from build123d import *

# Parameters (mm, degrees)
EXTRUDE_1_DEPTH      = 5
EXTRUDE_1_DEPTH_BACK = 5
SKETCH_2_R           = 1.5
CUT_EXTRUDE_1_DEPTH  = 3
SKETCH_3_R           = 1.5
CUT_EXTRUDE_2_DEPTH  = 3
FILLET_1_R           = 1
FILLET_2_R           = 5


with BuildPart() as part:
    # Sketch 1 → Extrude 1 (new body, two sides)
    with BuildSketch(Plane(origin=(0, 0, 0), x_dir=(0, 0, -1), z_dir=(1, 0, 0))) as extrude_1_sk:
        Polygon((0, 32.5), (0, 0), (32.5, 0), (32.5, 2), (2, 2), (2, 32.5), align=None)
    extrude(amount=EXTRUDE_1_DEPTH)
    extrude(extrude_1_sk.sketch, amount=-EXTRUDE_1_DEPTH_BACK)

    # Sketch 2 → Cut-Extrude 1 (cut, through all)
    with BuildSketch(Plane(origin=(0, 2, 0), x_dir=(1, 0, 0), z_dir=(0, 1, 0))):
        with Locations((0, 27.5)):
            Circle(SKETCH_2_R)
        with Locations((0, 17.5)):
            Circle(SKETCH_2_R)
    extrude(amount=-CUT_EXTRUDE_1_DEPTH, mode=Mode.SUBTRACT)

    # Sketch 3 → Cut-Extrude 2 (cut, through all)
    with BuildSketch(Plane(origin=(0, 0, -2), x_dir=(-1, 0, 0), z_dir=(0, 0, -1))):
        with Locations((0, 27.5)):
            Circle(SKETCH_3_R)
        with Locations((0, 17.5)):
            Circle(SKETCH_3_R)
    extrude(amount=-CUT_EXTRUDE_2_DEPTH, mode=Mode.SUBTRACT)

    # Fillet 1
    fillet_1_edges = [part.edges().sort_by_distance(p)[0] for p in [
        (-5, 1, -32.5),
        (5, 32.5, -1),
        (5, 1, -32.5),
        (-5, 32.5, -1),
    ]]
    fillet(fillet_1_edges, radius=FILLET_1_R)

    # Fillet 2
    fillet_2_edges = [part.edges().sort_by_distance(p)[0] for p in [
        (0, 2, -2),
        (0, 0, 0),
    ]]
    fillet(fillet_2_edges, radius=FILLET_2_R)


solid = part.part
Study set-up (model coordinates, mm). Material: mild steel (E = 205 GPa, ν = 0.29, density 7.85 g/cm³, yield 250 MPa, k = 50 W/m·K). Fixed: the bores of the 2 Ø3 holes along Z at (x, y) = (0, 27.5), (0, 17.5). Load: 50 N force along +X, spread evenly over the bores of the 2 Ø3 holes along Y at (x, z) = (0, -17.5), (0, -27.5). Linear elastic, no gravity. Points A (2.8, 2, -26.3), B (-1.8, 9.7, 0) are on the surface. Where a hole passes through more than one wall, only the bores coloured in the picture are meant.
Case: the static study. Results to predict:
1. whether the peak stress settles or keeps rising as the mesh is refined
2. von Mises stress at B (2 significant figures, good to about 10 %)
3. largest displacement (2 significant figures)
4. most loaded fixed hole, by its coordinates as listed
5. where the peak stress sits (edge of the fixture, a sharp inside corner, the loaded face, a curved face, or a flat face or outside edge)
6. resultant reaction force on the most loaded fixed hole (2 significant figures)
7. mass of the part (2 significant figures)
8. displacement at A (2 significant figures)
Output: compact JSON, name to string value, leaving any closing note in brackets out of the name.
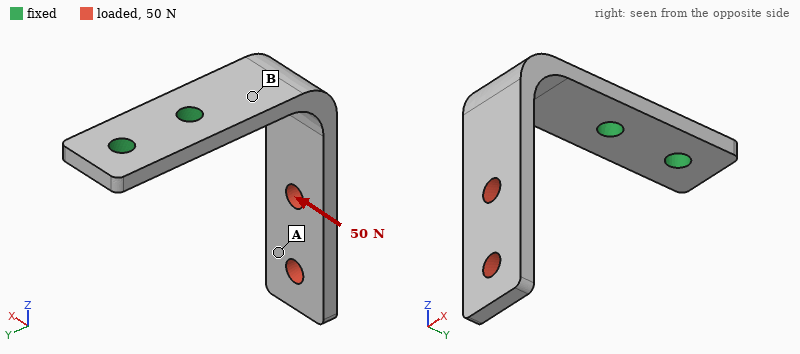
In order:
{"whether the peak stress settles or keeps rising as the mesh is refined": "keeps rising", "von Mises stress at B": "130 MPa", "largest displacement": "0.22 mm", "most loaded fixed hole, by its coordinates as listed": "(0, 17.5)", "where the peak stress sits": "edge of the fixture", "resultant reaction force on the most loaded fixed hole": "91 N", "mass of the part": "9.4 g", "displacement at A": "0.17 mm"}
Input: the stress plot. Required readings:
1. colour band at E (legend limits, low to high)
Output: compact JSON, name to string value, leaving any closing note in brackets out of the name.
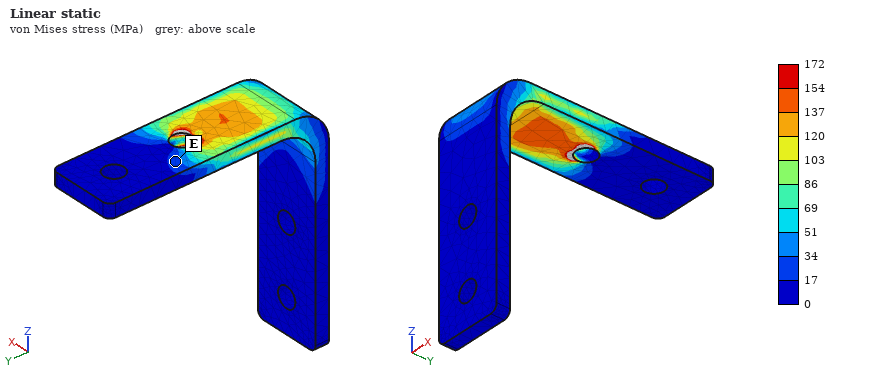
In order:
{"colour band at E": "17 to 34 MPa"}
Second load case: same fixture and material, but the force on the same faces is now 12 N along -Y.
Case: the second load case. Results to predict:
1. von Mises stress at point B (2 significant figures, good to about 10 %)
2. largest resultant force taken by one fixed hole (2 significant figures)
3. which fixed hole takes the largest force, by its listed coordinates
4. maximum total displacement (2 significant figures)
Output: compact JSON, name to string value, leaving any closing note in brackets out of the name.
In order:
{"von Mises stress at point B": "36 MPa", "largest resultant force taken by one fixed hole": "11 N", "which fixed hole takes the largest force, by its listed coordinates": "(0, 17.5)", "maximum total displacement": "0.11 mm"}
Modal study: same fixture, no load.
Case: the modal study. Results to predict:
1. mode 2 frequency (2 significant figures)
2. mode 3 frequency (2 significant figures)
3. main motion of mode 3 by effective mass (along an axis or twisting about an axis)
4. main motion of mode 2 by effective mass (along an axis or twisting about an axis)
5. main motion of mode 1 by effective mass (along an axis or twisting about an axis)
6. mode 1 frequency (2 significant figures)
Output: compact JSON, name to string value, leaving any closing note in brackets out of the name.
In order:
{"mode 2 frequency": "1600 Hz", "mode 3 frequency": "3700 Hz", "main motion of mode 3 by effective mass": "along Z", "main motion of mode 2 by effective mass": "along X", "main motion of mode 1 by effective mass": "along Y", "mode 1 frequency": "1100 Hz"}
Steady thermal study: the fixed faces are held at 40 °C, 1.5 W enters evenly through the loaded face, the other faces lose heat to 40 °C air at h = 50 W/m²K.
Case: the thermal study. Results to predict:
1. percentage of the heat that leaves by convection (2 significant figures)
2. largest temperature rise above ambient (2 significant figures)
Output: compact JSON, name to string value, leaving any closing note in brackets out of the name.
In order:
{"percentage of the heat that leaves by convection": "56 %", "largest temperature rise above ambient": "29 K"}
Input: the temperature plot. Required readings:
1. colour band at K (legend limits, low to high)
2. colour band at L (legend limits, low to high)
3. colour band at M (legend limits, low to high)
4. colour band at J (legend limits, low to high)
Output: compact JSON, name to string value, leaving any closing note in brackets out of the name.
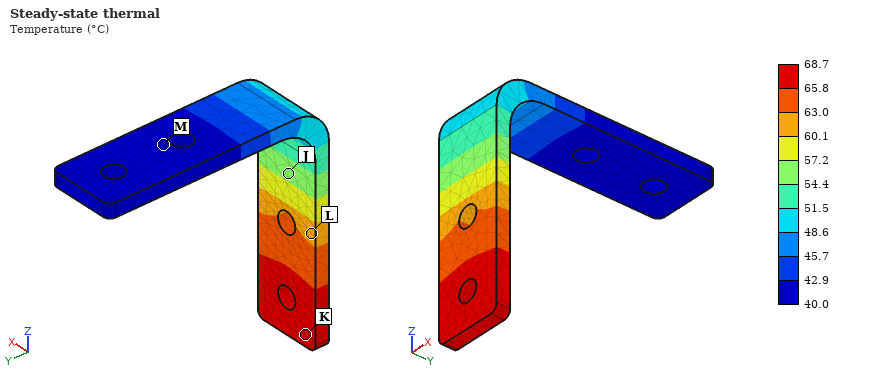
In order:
{"colour band at K": "65.8 to 68.7 °C", "colour band at L": "60.1 to 63.0 °C", "colour band at M": "40.0 to 42.9 °C", "colour band at J": "54.4 to 57.2 °C"}
